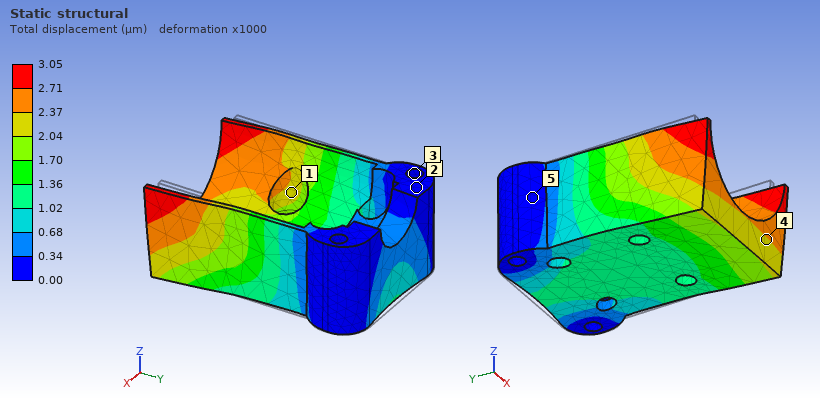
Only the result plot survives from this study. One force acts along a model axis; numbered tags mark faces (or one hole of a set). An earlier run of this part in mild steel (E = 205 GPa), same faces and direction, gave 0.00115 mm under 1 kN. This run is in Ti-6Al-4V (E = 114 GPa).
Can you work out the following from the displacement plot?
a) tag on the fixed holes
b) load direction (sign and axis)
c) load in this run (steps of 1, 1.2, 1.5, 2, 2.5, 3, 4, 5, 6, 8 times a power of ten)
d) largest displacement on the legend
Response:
3
-Y
1.5 kN
3.05 µm
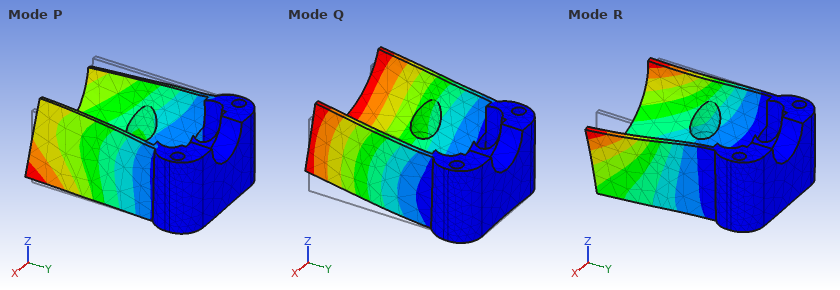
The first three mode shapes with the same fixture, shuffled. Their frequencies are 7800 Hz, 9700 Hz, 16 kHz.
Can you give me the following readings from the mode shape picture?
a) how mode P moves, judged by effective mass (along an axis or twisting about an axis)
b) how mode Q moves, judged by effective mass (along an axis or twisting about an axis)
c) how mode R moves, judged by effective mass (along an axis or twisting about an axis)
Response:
along X
along Z
along X
